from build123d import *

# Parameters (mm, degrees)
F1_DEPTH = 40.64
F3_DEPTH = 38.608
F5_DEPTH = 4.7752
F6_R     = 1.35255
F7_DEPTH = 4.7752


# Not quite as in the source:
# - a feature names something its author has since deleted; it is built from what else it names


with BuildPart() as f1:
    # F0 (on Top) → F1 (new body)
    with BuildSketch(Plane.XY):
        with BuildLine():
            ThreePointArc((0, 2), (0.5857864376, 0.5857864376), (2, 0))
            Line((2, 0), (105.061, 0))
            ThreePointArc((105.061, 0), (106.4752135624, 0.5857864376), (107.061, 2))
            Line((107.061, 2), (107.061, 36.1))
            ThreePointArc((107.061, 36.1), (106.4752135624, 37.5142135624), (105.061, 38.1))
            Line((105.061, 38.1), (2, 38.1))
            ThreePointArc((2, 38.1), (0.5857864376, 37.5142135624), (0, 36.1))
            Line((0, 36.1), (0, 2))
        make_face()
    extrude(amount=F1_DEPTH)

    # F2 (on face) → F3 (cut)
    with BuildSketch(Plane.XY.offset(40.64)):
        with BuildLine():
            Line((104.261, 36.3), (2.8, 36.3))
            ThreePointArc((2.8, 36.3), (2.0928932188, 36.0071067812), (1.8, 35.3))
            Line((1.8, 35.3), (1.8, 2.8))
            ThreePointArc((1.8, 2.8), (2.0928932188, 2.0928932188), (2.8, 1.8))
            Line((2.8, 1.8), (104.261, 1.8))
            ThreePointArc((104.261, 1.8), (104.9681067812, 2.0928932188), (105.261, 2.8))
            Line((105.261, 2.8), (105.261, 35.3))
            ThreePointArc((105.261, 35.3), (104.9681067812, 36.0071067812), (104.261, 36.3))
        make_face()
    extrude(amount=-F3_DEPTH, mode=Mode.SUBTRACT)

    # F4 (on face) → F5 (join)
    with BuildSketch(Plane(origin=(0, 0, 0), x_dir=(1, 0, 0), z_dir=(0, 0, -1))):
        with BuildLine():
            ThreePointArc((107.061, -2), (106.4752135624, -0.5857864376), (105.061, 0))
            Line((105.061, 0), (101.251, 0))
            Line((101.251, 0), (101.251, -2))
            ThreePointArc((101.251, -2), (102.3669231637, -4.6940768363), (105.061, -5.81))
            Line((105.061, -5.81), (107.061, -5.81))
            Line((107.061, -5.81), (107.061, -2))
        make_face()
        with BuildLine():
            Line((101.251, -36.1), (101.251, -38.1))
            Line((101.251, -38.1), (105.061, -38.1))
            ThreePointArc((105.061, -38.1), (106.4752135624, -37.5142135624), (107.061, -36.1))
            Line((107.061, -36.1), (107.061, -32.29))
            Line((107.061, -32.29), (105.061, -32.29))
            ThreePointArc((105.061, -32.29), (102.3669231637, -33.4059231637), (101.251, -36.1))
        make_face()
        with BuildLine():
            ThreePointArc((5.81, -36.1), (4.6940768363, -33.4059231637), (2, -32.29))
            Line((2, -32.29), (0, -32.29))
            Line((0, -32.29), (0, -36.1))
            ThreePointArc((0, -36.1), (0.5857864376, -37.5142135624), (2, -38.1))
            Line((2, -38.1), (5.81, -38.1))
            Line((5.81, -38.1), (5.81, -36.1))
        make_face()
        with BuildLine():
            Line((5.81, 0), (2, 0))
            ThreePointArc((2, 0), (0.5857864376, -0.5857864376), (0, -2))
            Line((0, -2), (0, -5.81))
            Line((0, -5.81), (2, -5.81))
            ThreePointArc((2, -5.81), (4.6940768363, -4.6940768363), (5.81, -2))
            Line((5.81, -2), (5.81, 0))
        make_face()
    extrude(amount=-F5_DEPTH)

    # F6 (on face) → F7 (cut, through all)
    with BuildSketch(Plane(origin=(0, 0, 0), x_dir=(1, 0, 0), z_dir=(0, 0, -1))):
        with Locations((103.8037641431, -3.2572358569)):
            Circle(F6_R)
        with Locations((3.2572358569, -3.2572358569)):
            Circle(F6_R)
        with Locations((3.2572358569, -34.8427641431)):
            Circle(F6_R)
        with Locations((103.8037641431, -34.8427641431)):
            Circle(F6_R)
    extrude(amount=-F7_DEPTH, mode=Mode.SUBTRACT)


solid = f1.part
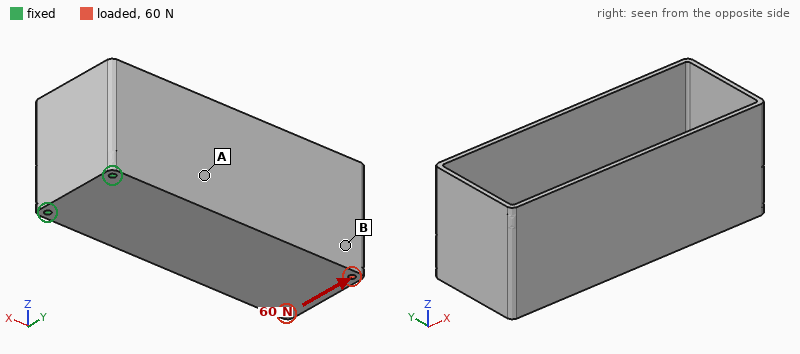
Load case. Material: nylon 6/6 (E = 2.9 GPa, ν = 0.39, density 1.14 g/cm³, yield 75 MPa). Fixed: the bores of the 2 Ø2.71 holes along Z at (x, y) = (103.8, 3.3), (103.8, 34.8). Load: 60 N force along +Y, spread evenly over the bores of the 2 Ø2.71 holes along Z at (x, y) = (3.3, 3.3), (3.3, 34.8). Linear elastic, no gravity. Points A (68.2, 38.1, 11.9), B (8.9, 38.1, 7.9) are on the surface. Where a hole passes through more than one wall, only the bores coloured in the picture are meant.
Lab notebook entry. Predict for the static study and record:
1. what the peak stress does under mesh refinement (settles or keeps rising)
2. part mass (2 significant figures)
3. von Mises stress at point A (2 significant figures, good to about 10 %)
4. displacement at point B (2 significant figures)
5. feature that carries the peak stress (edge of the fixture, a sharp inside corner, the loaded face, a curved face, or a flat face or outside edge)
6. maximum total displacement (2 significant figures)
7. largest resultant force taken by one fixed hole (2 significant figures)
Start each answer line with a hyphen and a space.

- keeps rising
- 32 g
- 2.3 MPa
- 0.68 mm
- edge of the fixture
- 1.3 mm
- 190 N
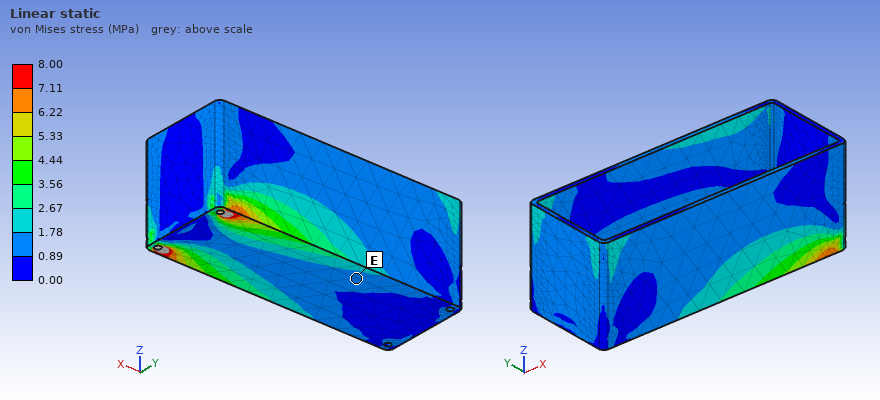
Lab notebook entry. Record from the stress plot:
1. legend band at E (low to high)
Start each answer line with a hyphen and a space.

- 0.89 to 1.78 MPa
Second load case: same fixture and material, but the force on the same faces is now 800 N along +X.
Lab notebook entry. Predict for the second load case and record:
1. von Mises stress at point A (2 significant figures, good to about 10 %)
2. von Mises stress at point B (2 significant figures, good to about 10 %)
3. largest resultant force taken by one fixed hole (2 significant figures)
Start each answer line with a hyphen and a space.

- 4.3 MPa
- 6.4 MPa
- 400 N
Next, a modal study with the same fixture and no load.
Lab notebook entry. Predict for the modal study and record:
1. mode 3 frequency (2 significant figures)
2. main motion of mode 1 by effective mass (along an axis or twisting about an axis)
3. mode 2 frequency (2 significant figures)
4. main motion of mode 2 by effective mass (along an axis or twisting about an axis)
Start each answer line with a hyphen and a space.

- 380 Hz
- along Z
- 170 Hz
- along Y
